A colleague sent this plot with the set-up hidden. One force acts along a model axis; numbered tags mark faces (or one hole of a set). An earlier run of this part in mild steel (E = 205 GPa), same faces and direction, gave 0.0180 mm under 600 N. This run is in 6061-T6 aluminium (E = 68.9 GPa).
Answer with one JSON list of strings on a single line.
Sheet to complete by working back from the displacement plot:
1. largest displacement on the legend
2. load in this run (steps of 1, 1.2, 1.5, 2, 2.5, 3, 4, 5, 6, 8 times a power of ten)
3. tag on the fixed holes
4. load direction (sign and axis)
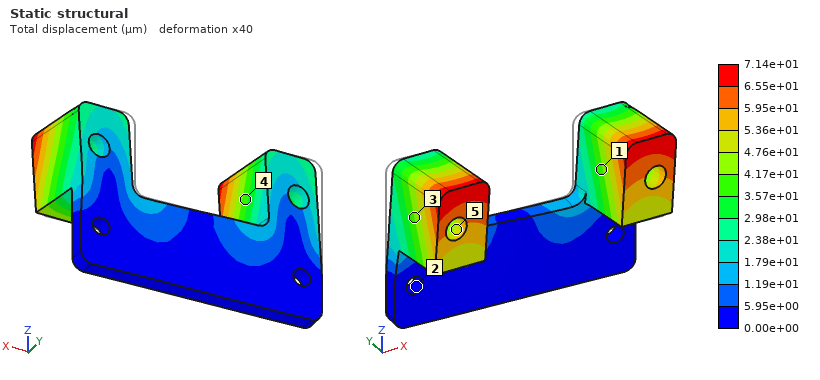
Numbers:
["7.14e+01 µm", "800 N", "2", "+X"]
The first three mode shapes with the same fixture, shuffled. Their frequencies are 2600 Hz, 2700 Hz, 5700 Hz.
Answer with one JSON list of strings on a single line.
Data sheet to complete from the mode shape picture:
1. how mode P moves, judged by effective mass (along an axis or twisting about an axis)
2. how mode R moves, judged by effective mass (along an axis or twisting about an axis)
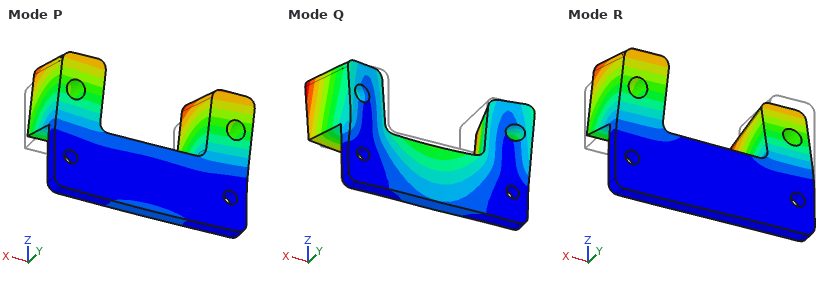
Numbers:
["along Y", "twisting about Z"]
